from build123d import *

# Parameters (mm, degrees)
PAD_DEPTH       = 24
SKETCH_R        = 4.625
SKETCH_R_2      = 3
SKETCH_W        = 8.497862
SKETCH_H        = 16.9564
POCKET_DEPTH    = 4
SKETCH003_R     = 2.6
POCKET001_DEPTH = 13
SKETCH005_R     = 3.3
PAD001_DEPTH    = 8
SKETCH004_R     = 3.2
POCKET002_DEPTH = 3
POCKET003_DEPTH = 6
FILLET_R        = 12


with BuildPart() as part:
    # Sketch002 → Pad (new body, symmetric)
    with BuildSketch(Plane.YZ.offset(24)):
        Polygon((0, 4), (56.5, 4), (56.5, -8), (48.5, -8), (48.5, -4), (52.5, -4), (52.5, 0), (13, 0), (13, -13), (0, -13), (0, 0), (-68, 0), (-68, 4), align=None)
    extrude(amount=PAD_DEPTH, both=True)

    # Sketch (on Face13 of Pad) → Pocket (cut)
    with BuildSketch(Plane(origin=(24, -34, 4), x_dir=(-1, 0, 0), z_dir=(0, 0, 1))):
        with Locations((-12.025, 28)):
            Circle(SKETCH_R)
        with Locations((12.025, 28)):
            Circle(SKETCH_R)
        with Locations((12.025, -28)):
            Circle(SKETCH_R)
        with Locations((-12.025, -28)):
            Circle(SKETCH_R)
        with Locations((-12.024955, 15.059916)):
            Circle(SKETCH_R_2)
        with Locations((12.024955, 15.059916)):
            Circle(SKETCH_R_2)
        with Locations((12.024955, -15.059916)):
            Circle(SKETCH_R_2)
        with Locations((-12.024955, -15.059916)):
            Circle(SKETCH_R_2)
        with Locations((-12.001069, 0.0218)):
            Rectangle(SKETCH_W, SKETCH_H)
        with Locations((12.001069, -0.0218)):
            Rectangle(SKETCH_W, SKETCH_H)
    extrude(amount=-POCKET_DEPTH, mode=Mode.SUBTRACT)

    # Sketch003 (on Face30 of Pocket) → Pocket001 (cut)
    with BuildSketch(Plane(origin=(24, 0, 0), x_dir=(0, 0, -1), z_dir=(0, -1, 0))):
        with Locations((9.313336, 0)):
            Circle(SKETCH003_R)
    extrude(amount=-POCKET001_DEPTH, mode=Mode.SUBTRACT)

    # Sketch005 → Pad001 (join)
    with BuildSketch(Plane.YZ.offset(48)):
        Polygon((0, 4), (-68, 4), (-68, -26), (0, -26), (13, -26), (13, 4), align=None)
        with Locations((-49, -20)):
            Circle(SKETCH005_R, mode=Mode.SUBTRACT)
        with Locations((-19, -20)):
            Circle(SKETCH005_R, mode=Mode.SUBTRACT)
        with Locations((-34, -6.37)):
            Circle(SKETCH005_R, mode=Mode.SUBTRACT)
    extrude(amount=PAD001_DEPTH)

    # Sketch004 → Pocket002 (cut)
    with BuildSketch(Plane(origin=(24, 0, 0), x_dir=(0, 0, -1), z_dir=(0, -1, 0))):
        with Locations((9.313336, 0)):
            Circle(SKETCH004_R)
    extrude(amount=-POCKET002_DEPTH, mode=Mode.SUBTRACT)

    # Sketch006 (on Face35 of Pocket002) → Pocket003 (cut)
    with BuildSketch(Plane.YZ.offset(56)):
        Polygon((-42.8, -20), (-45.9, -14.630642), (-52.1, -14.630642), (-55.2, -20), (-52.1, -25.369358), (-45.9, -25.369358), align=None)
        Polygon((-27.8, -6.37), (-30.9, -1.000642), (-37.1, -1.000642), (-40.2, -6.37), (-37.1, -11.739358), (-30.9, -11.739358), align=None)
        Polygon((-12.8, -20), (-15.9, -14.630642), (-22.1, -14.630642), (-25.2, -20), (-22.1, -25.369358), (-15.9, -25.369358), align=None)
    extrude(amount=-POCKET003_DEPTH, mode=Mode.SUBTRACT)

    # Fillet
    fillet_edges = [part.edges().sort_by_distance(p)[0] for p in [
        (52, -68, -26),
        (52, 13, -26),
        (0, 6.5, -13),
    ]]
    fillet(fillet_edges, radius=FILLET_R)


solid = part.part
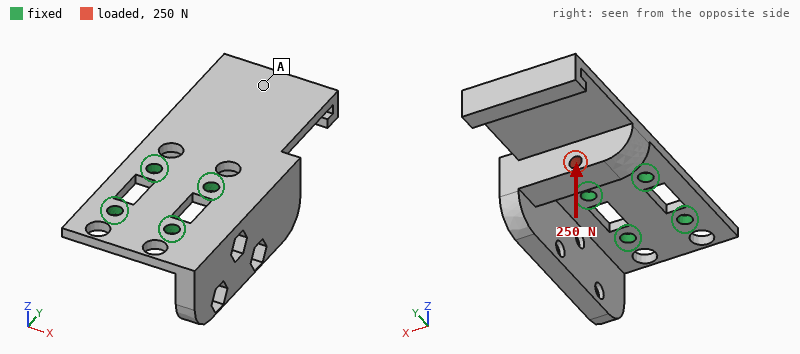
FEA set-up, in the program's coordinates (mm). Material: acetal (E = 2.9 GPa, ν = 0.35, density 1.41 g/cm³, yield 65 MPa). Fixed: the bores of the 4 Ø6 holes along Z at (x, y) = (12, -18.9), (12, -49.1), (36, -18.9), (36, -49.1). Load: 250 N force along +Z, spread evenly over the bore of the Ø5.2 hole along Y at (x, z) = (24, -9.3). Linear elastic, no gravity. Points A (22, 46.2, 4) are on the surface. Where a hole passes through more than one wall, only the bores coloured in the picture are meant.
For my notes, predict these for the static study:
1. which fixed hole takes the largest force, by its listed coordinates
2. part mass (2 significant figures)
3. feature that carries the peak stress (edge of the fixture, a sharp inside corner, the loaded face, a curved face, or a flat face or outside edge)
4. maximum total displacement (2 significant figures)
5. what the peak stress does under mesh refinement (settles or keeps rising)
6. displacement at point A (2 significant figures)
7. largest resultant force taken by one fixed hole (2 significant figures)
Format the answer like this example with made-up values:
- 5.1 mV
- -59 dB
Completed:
- (36, -18.9)
- 67 g
- edge of the fixture
- 1.6 mm
- keeps rising
- 1.2 mm
- 260 N
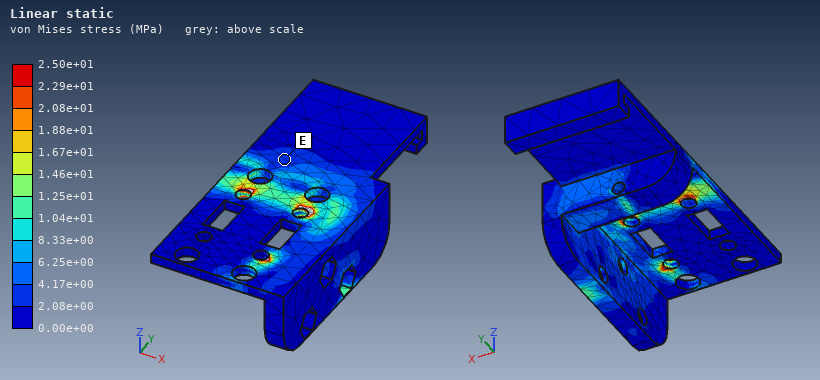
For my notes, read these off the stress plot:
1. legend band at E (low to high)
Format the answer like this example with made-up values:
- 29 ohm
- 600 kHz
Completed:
- 2.08e+00 to 4.17e+00 MPa
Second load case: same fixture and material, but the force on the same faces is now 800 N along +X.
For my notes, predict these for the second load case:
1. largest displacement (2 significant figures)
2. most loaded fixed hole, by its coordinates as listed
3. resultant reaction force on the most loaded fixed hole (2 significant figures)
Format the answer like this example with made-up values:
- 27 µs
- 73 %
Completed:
- 1.3 mm
- (36, -18.9)
- 730 N
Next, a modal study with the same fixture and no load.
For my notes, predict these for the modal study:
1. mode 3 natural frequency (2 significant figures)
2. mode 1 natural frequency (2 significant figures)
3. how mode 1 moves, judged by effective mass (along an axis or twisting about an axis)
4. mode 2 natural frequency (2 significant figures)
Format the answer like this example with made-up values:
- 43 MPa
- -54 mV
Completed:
- 760 Hz
- 250 Hz
- along Z
- 560 Hz
